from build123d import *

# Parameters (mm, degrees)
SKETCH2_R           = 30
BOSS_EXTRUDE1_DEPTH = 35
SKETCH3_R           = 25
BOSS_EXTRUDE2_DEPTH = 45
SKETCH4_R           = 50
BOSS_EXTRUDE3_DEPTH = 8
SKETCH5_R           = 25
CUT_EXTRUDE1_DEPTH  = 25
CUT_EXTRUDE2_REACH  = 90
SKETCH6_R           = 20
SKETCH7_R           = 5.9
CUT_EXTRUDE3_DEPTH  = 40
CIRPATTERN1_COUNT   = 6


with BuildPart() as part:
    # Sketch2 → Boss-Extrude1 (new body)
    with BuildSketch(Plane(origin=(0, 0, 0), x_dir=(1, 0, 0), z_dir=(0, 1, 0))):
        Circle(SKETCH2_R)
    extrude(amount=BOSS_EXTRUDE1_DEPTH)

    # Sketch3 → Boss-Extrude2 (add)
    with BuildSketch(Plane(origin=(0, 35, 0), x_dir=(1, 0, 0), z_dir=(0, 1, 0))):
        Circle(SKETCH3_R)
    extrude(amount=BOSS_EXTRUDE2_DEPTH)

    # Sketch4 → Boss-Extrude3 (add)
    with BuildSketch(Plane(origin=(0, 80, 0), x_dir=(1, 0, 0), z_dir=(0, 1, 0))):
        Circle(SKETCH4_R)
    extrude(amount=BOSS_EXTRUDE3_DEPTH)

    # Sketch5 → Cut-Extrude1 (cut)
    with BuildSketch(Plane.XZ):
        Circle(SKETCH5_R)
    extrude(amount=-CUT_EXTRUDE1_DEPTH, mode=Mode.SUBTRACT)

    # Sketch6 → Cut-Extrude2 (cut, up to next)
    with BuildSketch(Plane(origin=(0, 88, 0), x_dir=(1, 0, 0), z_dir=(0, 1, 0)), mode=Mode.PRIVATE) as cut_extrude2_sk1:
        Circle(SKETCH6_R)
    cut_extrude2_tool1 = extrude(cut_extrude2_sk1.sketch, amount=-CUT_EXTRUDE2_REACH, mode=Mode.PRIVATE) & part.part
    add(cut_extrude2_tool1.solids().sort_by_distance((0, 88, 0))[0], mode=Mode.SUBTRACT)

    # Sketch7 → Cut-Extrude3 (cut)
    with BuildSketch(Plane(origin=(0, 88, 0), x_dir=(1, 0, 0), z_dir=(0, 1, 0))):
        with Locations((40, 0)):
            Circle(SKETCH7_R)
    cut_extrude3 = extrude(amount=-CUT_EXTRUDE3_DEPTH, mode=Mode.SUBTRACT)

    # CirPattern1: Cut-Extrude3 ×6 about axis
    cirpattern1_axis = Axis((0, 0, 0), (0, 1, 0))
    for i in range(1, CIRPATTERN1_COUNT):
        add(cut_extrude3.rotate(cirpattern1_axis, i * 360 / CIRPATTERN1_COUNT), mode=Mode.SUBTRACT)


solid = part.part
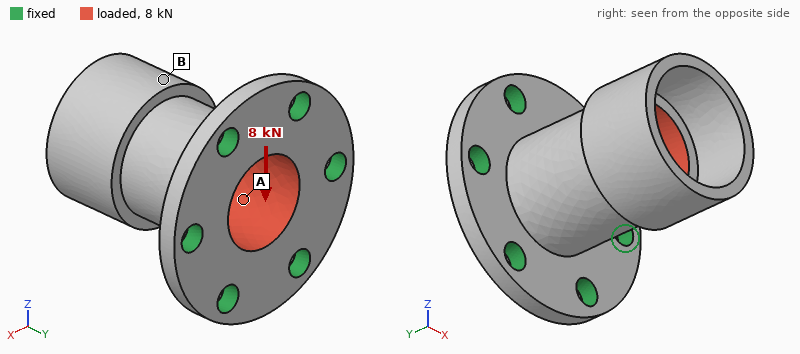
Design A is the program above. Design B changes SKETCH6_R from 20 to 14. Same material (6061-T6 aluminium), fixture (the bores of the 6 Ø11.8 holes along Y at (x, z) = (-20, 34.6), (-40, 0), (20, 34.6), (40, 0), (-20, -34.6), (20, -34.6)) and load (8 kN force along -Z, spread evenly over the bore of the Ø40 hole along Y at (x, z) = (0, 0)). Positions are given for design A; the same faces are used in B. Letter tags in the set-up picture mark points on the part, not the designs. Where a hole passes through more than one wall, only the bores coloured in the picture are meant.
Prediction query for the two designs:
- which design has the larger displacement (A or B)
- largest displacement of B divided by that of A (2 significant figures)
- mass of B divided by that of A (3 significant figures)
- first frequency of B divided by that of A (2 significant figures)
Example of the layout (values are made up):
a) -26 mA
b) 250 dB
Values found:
a) A
b) 0.70
c) 1.35
d) 1.1
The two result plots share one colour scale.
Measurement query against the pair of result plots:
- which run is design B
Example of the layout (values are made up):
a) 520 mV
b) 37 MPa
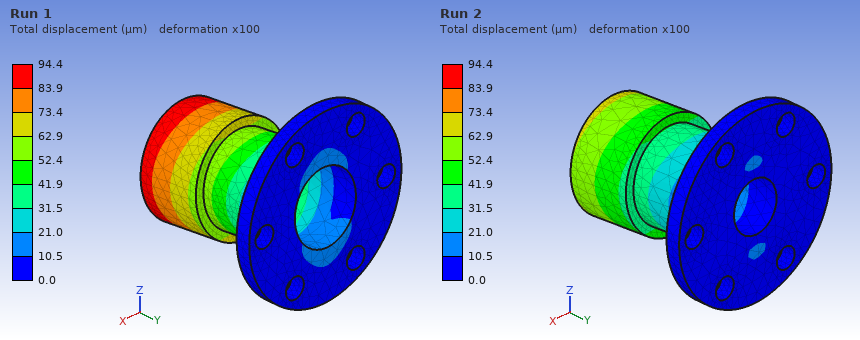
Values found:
a) Run 2
